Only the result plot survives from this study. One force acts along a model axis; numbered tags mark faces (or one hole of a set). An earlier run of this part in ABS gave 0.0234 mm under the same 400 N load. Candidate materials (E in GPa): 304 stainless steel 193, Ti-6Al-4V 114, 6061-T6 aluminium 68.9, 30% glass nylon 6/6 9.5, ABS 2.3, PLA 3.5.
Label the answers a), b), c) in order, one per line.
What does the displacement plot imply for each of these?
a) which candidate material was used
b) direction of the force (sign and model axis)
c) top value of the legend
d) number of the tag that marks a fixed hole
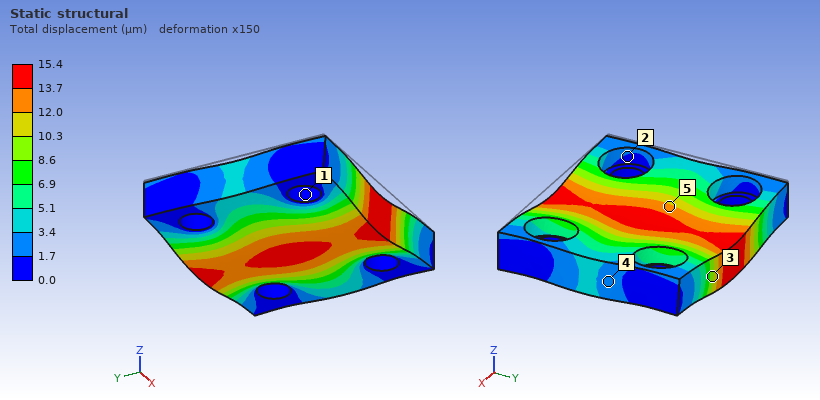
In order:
a) PLA
b) -Z
c) 15.4 µm
d) 1
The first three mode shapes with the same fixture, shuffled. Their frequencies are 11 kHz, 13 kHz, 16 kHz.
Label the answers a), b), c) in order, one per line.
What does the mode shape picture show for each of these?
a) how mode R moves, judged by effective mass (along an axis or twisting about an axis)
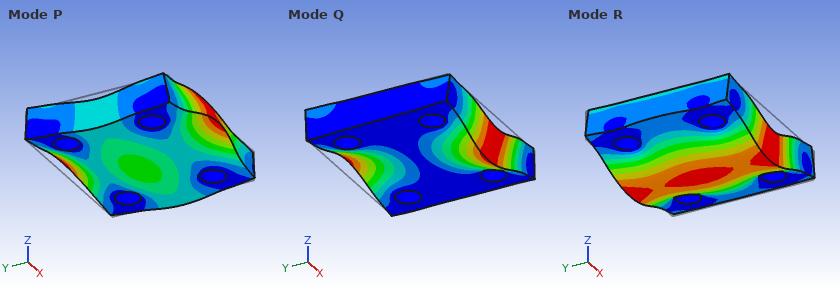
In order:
a) along Z
